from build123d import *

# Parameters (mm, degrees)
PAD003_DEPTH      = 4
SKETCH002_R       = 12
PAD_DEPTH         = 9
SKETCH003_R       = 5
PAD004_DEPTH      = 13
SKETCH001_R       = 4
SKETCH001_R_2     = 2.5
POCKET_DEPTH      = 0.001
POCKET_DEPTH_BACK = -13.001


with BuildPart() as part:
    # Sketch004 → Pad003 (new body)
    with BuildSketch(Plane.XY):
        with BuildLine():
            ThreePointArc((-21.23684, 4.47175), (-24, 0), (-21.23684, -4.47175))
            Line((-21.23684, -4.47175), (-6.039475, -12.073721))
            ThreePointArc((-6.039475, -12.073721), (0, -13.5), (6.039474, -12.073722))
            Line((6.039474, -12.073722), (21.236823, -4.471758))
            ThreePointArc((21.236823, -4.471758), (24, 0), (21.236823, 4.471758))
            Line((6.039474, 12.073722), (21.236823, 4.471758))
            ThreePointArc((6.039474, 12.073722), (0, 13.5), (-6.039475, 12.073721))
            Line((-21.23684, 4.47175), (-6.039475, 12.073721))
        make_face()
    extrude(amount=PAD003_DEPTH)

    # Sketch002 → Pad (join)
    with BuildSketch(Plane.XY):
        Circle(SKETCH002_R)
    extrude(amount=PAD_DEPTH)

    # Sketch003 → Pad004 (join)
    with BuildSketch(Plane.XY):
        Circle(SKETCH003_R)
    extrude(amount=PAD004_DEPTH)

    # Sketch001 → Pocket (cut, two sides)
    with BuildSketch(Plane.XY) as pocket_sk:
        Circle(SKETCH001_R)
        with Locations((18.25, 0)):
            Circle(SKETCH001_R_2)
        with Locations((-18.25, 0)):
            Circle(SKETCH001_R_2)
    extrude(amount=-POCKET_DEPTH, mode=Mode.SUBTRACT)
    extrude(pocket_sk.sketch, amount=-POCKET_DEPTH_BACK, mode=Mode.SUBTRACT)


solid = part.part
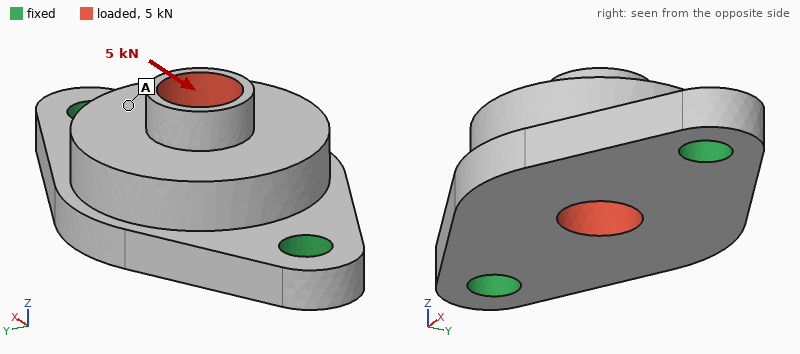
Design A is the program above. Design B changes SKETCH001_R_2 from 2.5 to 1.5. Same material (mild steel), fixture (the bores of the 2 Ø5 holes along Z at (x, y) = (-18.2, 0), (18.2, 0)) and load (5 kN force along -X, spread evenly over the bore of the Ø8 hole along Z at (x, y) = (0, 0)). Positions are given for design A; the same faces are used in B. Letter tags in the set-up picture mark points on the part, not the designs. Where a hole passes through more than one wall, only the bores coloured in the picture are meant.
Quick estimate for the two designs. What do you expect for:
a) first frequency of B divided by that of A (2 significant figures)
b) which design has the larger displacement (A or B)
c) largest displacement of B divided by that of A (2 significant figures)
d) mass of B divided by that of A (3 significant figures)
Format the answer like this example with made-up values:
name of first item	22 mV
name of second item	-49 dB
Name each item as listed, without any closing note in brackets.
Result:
first frequency of B divided by that of A	0.85
which design has the larger displacement	B
largest displacement of B divided by that of A	1.1
mass of B divided by that of A	1.02
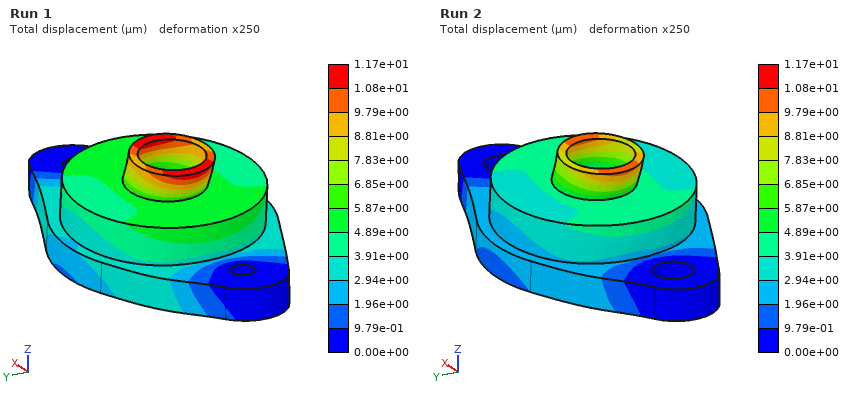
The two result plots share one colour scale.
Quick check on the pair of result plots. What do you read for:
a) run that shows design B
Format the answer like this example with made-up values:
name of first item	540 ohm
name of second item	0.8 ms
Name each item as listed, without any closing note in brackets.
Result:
run that shows design B	Run 1
